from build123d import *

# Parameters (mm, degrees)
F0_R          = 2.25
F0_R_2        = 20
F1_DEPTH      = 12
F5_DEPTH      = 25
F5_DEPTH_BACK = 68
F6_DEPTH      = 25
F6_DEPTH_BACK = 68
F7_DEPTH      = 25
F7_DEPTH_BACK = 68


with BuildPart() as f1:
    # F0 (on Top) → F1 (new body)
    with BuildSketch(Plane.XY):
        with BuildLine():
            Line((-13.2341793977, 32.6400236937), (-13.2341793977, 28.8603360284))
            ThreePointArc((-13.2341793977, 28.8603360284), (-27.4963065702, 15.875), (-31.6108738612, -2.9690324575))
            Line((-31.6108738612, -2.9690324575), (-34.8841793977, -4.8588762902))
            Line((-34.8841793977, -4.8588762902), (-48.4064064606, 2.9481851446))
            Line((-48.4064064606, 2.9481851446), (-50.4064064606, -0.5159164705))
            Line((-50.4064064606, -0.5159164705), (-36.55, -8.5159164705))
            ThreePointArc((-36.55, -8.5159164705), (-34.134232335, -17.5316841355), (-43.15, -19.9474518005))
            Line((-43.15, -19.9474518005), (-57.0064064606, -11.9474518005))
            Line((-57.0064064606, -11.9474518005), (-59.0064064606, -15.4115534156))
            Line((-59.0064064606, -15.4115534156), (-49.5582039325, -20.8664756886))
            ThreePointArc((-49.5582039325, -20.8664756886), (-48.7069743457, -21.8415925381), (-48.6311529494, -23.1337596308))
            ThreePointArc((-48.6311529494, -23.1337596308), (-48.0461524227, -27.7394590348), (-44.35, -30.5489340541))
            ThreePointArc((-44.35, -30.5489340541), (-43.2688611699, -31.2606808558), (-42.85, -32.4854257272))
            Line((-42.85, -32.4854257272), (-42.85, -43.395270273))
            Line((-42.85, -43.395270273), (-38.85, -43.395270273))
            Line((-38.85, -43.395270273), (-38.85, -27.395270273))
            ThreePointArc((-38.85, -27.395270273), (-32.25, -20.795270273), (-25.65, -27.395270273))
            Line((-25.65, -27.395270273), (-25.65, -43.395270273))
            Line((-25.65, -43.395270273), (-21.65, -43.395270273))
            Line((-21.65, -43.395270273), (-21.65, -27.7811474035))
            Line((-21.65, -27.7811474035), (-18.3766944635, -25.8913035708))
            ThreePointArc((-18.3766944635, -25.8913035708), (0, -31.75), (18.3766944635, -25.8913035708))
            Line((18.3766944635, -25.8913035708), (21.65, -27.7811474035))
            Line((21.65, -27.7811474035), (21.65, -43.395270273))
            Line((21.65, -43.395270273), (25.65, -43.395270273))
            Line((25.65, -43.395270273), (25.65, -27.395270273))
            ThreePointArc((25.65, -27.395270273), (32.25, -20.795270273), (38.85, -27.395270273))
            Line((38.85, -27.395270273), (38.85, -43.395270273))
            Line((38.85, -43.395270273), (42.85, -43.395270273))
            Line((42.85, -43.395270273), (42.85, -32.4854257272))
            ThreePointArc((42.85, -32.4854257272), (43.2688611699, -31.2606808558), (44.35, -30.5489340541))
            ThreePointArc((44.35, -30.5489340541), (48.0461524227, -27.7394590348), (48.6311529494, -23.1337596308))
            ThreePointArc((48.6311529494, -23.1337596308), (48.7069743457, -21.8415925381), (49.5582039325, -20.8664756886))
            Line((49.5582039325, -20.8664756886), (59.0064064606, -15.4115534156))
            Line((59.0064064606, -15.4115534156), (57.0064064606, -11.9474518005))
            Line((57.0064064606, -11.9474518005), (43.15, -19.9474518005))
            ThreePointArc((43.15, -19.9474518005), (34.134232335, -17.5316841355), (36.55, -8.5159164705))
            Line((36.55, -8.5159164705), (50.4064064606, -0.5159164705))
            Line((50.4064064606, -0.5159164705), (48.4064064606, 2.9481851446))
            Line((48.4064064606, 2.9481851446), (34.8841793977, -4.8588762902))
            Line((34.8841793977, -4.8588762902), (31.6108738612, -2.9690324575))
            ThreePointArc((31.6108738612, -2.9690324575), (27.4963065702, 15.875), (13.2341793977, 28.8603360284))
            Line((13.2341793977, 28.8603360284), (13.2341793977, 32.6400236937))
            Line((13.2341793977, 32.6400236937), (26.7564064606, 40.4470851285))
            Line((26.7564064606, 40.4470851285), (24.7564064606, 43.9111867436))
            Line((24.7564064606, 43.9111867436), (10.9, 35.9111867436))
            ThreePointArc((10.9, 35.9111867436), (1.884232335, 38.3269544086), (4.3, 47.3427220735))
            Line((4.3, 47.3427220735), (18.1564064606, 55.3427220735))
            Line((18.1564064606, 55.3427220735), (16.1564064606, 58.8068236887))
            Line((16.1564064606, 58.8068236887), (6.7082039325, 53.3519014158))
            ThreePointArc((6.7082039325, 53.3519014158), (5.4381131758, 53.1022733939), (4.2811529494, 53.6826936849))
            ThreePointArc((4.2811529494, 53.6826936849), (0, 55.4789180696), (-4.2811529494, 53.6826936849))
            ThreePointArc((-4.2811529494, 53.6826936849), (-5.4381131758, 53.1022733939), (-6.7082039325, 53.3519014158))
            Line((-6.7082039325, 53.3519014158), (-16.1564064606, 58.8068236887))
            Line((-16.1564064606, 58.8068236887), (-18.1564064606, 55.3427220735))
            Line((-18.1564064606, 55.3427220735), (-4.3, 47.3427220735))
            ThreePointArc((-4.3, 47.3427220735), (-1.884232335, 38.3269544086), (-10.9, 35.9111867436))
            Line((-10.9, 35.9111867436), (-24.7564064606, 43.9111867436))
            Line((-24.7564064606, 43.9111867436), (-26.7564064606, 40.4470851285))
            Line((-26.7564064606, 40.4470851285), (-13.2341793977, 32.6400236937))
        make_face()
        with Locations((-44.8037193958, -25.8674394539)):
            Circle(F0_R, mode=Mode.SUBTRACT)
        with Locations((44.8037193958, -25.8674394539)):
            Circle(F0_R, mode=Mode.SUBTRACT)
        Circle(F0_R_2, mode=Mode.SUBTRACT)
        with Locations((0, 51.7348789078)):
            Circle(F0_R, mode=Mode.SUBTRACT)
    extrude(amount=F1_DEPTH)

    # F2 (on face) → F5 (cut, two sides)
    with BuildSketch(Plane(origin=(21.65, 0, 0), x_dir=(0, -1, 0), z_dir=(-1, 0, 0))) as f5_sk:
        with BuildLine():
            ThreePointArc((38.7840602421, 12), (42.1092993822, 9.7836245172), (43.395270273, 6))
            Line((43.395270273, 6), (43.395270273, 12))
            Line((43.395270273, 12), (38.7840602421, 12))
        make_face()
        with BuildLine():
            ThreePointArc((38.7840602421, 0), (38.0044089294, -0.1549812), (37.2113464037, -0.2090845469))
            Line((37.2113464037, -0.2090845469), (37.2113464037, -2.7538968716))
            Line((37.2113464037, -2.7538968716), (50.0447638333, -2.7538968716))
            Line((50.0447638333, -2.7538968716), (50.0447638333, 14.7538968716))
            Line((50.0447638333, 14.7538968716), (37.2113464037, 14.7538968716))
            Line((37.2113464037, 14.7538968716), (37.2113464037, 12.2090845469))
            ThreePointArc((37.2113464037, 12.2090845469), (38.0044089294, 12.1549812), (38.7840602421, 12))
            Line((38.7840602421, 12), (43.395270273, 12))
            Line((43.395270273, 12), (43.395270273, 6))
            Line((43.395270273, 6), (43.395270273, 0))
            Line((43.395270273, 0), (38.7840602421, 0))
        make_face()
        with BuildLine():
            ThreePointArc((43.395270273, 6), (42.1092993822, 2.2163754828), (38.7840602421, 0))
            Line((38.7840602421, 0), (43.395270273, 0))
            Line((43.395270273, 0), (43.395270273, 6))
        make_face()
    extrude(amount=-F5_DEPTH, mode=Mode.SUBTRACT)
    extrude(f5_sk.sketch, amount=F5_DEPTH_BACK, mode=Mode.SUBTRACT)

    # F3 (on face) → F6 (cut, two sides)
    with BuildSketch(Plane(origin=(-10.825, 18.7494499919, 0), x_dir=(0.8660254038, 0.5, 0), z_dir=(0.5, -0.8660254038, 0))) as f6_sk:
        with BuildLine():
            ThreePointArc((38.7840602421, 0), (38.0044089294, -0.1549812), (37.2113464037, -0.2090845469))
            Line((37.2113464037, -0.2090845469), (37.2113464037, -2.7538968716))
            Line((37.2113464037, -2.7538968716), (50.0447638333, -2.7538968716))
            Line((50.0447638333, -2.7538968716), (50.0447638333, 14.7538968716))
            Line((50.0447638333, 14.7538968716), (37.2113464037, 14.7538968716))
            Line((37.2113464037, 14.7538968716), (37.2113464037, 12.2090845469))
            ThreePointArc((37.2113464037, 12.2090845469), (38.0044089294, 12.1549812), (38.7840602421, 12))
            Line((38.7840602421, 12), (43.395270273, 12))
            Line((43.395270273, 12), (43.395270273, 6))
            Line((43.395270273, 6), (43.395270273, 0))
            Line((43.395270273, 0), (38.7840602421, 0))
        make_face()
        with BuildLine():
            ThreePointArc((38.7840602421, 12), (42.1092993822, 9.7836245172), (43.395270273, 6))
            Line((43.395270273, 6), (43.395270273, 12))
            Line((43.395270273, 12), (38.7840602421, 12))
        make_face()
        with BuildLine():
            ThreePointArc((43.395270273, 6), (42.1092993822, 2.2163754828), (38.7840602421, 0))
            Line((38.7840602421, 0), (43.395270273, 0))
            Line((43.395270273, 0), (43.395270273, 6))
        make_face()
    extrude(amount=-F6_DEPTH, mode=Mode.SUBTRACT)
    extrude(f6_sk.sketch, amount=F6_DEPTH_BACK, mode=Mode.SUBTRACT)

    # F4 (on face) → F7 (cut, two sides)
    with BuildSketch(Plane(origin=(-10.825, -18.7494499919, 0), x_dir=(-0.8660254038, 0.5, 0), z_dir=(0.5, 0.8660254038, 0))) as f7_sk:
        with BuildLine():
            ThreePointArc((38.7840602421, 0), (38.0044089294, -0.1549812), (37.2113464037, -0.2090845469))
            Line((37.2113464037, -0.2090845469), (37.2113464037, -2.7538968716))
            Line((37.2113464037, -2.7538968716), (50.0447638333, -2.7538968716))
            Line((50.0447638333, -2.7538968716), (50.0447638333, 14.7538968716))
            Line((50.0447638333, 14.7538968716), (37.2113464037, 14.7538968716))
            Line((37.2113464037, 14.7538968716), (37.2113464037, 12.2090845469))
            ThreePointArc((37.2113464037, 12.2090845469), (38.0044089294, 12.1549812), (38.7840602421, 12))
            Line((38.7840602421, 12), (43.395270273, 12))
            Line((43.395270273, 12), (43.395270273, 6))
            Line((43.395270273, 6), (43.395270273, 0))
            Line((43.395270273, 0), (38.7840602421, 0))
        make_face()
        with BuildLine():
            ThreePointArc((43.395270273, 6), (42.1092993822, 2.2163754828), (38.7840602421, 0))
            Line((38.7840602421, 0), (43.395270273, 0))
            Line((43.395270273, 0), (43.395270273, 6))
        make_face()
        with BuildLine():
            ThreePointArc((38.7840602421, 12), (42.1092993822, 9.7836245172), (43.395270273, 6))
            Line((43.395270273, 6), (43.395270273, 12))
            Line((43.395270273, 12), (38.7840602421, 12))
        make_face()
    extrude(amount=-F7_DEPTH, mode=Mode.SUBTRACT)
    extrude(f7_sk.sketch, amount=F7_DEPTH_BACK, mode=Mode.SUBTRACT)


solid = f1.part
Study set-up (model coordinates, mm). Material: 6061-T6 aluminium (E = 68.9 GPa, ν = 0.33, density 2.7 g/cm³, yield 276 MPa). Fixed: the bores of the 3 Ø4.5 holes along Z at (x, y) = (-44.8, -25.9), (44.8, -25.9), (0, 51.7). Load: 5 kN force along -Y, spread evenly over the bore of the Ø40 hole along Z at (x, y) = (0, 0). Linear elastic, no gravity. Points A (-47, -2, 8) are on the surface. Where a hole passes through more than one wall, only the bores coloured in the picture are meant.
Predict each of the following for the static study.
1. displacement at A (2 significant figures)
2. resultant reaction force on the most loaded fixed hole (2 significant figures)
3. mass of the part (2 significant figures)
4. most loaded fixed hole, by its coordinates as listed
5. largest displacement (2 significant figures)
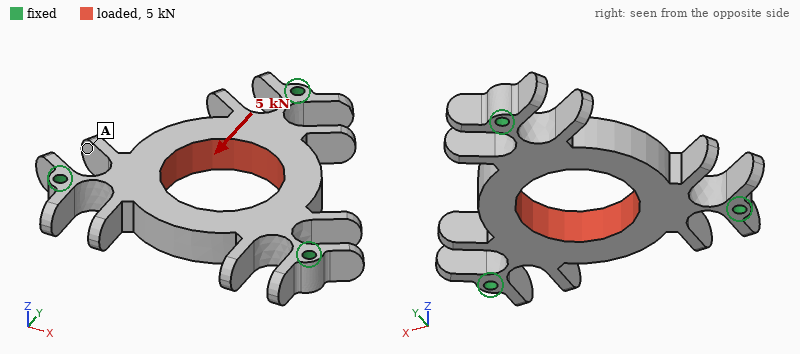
29 µm
2.7 kN
100 g
(0, 51.7)
58 µm
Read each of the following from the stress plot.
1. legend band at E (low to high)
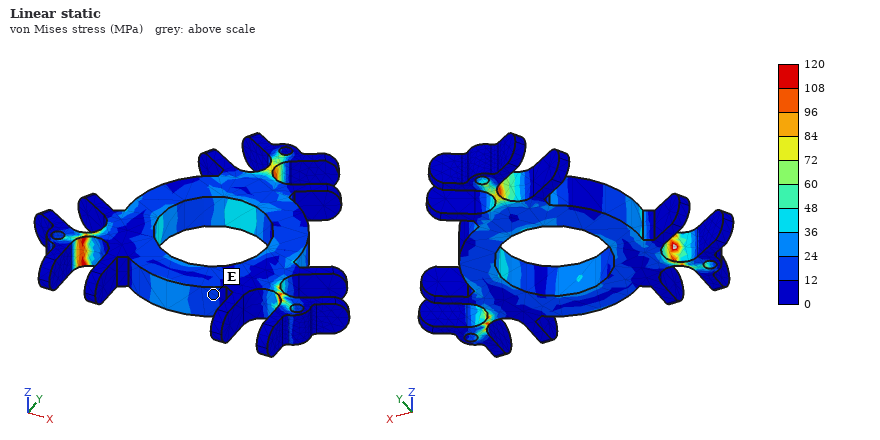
12 to 24 MPa
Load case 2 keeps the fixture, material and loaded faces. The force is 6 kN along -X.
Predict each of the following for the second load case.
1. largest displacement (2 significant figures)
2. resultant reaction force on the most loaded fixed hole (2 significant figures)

65 µm
2.8 kN
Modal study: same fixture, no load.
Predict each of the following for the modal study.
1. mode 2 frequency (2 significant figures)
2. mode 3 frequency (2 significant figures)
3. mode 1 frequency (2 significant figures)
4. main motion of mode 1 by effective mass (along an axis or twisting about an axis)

4400 Hz
4400 Hz
4200 Hz
along Z
